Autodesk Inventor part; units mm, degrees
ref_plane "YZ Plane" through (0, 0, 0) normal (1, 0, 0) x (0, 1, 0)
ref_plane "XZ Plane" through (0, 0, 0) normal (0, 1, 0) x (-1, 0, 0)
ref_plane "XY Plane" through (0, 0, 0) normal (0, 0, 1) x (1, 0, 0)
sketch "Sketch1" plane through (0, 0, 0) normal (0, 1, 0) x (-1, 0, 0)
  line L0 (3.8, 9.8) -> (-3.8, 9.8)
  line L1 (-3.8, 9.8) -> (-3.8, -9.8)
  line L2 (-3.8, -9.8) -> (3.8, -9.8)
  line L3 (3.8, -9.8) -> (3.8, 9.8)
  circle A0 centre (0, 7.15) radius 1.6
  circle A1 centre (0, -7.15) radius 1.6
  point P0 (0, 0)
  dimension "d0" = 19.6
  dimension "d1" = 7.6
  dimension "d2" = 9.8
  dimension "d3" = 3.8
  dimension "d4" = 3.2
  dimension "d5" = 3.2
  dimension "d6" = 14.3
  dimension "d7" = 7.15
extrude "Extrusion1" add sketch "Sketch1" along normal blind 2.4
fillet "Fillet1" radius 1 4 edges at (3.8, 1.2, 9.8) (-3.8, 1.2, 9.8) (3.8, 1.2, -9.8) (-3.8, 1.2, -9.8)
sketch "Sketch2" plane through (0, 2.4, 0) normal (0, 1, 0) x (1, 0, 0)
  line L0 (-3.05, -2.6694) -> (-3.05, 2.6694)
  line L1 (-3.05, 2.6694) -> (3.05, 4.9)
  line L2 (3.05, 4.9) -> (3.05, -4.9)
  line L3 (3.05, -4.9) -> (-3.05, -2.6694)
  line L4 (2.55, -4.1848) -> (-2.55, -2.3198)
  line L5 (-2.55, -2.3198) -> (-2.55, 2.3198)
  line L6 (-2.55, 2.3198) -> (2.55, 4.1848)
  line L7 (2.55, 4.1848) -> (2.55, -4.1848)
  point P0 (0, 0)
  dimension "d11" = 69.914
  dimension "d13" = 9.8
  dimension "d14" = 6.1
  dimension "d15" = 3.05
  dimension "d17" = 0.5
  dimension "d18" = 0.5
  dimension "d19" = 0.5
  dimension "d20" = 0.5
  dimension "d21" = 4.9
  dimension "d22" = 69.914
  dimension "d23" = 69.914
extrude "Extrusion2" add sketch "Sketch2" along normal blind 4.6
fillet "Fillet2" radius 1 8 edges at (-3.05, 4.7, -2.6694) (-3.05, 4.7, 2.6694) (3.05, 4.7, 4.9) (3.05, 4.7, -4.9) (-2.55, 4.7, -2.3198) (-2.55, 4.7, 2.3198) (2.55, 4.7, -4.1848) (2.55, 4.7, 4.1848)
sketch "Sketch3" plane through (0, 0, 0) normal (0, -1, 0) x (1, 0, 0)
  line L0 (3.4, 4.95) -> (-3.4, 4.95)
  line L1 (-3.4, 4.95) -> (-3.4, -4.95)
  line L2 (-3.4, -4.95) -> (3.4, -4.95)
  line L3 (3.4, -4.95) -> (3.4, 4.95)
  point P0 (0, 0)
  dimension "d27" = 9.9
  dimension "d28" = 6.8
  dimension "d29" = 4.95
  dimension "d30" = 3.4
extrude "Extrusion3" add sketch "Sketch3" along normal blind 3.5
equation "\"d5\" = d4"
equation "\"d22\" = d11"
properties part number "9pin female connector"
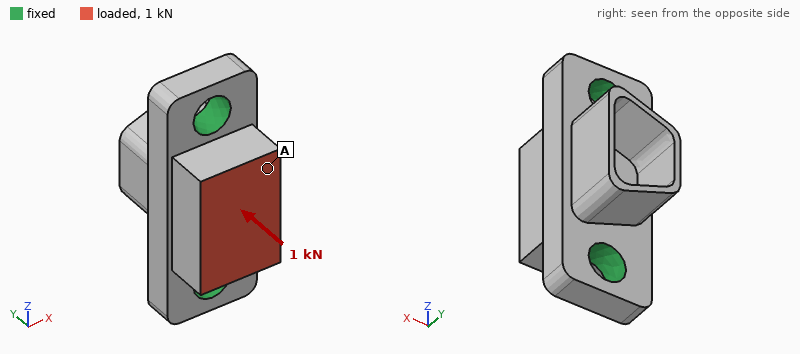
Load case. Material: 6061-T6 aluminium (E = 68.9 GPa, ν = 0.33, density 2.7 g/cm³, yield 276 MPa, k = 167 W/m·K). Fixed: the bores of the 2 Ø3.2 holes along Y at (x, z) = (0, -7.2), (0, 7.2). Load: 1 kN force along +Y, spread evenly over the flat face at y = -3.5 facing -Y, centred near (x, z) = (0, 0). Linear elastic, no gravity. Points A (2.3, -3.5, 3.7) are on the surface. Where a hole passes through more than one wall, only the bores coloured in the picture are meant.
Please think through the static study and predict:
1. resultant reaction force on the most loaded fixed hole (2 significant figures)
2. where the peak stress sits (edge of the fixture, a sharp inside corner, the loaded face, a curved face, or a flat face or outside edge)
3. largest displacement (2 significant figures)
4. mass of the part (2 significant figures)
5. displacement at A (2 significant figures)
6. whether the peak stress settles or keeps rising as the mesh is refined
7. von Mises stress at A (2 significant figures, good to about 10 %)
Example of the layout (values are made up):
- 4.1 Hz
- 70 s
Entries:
- 530 N
- edge of the fixture
- 5.7 µm
- 1.7 g
- 4.6 µm
- keeps rising
- 15 MPa
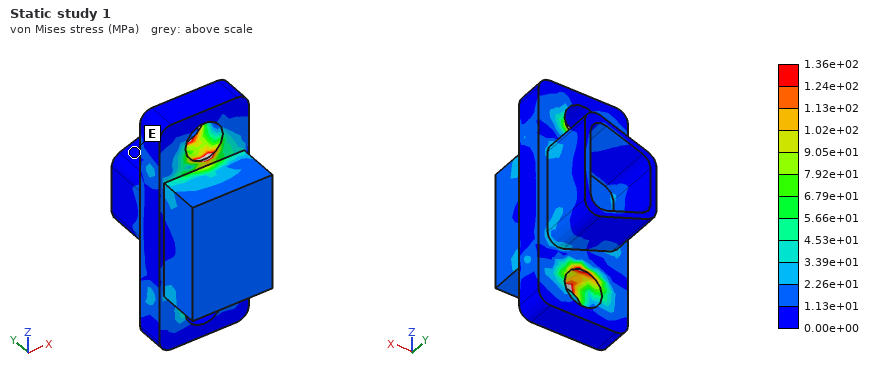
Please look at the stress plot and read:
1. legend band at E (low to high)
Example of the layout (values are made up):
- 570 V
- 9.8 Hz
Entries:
- 0.00e+00 to 1.13e+01 MPa
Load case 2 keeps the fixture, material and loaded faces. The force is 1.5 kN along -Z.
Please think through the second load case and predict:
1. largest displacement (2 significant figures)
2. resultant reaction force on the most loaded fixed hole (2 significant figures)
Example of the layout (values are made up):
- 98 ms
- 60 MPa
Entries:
- 11 µm
- 980 N
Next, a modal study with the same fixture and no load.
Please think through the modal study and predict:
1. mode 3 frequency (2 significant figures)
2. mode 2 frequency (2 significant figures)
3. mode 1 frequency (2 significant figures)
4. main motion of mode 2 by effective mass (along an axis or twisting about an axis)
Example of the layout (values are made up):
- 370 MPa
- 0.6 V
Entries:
- 63 kHz
- 46 kHz
- 39 kHz
- along X
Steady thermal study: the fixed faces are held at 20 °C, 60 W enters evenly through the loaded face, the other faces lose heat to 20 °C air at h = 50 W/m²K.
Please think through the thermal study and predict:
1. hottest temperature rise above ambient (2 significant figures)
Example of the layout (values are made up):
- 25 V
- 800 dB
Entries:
- 48 K
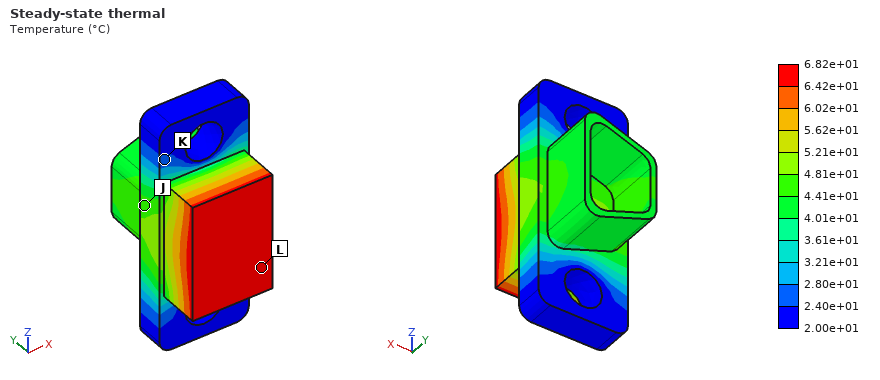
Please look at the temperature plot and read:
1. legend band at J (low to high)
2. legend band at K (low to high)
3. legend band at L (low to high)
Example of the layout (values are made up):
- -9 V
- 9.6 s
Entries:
- 4.41e+01 to 4.81e+01 °C
- 2.40e+01 to 2.80e+01 °C
- 6.42e+01 to 6.82e+01 °C
